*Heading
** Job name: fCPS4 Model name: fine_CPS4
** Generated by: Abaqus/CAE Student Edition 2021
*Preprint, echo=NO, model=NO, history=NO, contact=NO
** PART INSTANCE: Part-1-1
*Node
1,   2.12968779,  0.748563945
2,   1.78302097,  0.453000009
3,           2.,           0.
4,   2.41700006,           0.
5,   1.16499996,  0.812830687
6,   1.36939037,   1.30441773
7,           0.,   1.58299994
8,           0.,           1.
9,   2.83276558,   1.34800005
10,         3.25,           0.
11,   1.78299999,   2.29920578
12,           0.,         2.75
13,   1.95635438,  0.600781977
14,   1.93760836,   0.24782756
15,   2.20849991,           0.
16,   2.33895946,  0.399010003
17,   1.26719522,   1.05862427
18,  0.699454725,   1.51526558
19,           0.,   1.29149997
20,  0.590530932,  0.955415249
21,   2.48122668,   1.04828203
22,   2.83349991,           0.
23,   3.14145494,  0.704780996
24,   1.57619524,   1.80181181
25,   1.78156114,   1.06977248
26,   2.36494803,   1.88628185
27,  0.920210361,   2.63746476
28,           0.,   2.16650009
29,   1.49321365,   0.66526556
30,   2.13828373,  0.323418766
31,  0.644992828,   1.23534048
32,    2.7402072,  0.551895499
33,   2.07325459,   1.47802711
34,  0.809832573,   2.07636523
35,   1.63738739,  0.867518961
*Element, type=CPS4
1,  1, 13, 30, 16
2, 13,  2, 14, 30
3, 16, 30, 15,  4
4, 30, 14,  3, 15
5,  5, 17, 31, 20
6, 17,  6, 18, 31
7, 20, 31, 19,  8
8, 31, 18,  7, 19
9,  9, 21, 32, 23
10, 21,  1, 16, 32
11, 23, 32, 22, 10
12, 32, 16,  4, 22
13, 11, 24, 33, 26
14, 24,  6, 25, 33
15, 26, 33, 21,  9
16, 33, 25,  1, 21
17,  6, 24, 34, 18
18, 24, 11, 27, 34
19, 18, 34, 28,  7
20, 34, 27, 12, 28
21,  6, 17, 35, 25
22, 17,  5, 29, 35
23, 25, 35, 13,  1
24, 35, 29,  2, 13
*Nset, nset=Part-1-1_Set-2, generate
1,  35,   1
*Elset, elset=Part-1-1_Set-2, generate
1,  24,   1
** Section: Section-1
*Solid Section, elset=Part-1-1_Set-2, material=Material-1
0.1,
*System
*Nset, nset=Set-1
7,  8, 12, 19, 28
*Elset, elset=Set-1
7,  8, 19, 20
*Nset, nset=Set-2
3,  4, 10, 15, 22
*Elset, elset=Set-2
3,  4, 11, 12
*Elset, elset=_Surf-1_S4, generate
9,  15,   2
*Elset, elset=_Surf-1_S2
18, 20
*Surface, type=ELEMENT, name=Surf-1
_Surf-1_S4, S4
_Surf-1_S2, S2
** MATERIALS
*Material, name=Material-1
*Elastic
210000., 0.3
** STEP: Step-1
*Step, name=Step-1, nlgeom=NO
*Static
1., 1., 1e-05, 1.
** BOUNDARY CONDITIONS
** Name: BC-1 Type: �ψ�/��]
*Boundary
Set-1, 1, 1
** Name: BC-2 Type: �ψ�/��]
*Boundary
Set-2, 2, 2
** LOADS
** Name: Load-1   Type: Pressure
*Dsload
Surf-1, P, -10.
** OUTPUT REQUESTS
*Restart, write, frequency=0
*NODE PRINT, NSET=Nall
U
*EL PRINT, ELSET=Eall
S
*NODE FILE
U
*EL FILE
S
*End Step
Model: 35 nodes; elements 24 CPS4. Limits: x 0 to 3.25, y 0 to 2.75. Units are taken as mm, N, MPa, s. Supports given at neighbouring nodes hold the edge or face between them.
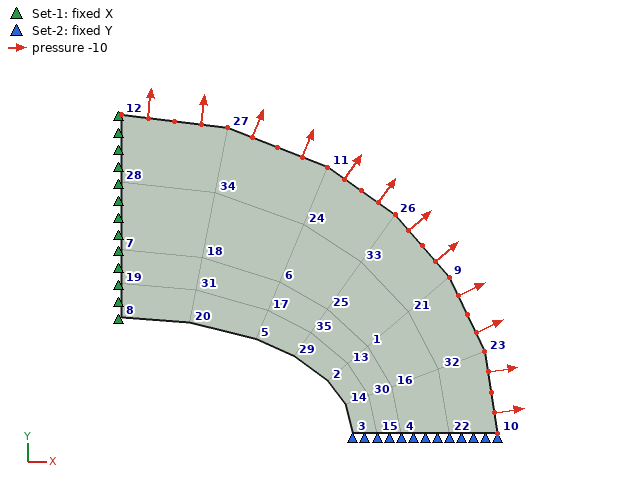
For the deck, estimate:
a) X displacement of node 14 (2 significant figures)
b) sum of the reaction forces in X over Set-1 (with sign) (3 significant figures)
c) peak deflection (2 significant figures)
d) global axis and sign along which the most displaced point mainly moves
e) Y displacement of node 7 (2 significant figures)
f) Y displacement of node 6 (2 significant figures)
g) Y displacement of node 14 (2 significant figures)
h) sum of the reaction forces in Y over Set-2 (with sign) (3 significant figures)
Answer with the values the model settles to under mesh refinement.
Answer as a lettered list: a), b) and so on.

a) -9.8e-05 mm
b) -2.75 N
c) 5.5e-04 mm
d) +Y
e) 5.5e-04 mm
f) 3.8e-04 mm
g) 1.1e-04 mm
h) -3.25 N
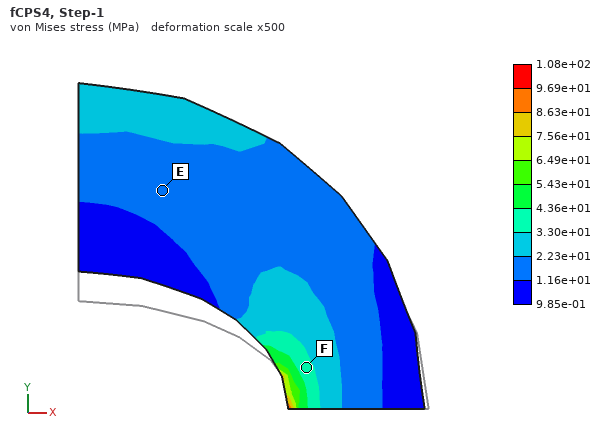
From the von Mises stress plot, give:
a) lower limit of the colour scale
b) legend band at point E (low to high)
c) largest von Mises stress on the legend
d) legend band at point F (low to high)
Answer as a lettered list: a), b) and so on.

a) 9.85e-01 MPa
b) 1.16e+01 to 2.23e+01 MPa
c) 1.08e+02 MPa
d) 3.30e+01 to 4.36e+01 MPa
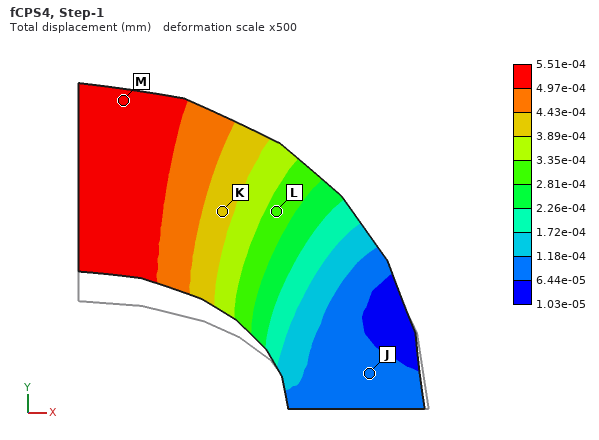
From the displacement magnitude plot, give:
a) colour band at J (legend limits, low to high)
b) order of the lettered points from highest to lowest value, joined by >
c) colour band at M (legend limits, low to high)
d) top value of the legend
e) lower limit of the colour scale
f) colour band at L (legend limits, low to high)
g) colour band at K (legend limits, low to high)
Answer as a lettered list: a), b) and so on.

a) 6.44e-05 to 1.18e-04 mm
b) M > K > L > J
c) 4.97e-04 to 5.51e-04 mm
d) 5.51e-04 mm
e) 1.03e-05 mm
f) 2.81e-04 to 3.35e-04 mm
g) 3.89e-04 to 4.43e-04 mm
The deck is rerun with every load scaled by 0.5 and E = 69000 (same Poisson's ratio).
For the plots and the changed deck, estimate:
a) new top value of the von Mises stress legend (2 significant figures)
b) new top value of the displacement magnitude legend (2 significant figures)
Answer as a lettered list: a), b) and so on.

a) 54 MPa
b) 8.4e-04 mm
